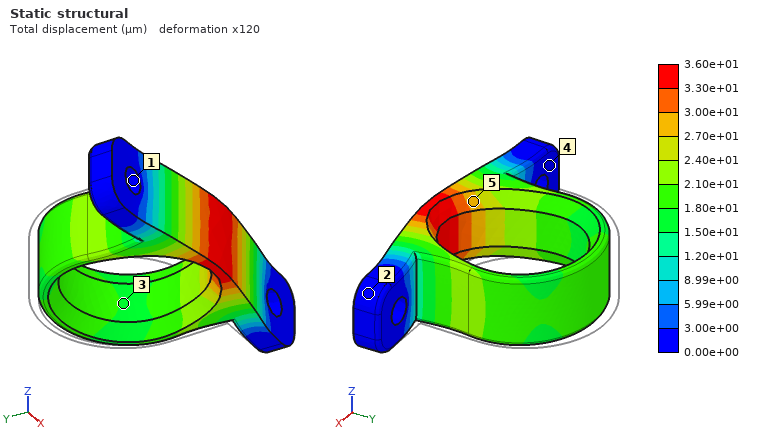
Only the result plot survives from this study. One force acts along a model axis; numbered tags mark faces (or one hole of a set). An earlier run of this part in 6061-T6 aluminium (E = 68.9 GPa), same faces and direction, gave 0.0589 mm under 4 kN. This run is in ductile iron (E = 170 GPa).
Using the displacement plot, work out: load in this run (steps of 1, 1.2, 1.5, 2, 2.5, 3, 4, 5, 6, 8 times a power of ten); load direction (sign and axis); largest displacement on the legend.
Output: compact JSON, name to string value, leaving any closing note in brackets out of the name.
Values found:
{"load in this run": "6 kN", "load direction": "-Y", "largest displacement on the legend": "3.60e+01 µm"}
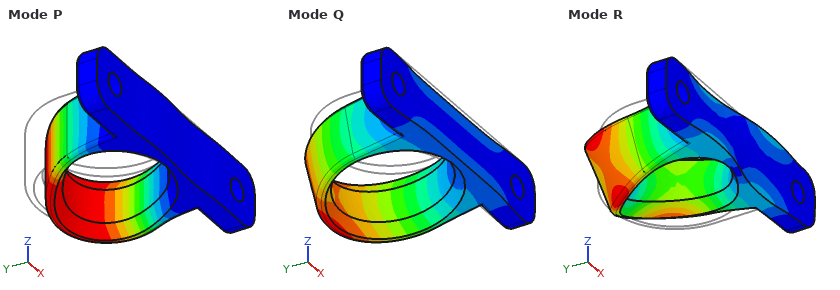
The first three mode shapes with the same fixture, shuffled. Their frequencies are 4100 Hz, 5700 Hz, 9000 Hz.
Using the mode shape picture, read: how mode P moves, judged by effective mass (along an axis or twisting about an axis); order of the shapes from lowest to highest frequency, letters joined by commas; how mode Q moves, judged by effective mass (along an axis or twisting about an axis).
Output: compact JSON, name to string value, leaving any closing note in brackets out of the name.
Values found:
{"how mode P moves, judged by effective mass": "along X", "order of the shapes from lowest to highest frequency, letters joined by commas": "Q, P, R", "how mode Q moves, judged by effective mass": "along Z"}
